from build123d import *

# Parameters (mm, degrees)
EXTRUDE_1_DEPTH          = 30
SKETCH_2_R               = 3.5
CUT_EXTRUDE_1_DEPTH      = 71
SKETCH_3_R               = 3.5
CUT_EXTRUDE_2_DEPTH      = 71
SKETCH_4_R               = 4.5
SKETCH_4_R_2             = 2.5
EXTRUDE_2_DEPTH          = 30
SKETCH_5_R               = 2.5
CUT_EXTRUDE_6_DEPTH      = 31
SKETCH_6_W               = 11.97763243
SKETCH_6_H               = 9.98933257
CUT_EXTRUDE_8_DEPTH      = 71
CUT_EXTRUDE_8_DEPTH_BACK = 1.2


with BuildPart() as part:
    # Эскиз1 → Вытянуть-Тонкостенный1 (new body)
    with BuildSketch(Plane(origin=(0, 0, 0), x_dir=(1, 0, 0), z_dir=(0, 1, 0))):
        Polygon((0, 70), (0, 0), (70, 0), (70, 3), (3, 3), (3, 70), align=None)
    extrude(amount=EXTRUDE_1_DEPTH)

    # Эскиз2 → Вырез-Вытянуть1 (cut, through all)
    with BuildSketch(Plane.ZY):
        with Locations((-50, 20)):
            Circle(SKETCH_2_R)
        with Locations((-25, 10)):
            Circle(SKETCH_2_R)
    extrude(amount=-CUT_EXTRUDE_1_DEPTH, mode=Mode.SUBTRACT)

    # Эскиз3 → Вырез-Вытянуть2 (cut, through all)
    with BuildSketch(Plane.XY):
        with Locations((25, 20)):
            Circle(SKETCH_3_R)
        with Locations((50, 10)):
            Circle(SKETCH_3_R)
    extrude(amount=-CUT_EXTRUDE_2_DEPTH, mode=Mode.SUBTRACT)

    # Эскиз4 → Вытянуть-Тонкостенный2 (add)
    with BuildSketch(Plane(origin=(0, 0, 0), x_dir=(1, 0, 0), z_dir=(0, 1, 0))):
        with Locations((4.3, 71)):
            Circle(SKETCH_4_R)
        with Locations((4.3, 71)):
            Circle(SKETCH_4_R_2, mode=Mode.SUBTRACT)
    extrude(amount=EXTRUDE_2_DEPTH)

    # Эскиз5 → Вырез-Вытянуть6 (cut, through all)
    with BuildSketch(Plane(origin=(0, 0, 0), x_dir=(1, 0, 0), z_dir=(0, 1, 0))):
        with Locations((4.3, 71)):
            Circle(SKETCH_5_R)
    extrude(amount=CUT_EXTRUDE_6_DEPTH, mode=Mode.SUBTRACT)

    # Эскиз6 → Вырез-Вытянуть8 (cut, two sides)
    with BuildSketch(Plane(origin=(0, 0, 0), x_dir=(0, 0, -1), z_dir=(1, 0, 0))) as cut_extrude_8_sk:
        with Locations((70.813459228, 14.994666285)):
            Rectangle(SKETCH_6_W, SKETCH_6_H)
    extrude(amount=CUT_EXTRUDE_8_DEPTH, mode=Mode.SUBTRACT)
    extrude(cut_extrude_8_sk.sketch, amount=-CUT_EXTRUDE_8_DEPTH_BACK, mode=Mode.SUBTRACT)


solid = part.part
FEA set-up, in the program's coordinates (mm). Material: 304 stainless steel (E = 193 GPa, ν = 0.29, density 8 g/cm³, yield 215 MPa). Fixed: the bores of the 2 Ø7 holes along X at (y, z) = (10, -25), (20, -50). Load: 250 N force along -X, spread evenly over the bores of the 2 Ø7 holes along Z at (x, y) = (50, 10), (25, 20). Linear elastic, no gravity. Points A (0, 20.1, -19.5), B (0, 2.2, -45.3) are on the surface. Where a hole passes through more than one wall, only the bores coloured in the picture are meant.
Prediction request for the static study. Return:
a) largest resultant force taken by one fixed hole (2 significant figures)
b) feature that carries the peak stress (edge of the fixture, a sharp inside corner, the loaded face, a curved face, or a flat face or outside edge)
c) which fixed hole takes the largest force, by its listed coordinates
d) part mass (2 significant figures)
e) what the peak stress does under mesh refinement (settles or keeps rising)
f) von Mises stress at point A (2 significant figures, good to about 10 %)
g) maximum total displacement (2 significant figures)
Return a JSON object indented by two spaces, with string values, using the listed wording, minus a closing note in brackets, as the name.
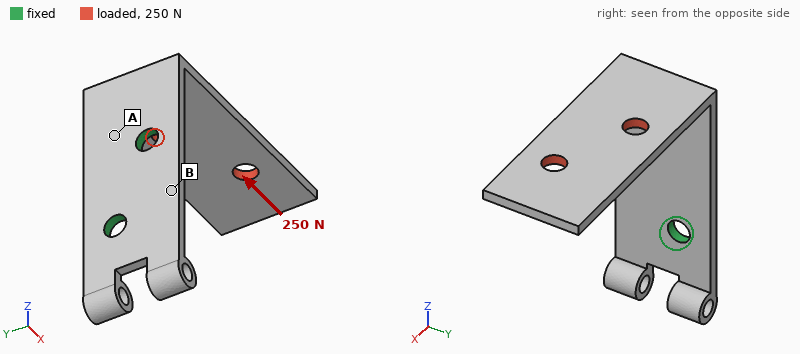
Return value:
{
  "largest resultant force taken by one fixed hole": "290 N",
  "feature that carries the peak stress": "edge of the fixture",
  "which fixed hole takes the largest force, by its listed coordinates": "(10, -25)",
  "part mass": "100 g",
  "what the peak stress does under mesh refinement": "keeps rising",
  "von Mises stress at point A": "74 MPa",
  "maximum total displacement": "0.34 mm"
}
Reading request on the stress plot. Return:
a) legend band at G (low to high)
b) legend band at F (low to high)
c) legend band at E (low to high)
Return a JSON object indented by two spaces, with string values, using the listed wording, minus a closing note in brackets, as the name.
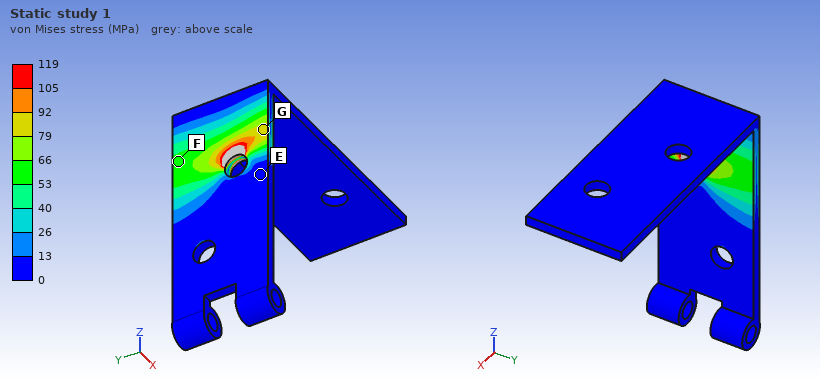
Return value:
{
  "legend band at G": "79 to 92 MPa",
  "legend band at F": "53 to 66 MPa",
  "legend band at E": "0 to 13 MPa"
}
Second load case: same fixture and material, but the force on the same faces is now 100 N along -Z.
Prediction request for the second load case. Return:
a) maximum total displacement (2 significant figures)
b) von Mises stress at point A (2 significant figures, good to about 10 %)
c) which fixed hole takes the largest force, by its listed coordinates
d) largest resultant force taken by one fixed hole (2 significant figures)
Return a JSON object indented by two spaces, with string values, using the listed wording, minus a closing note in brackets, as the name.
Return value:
{
  "maximum total displacement": "0.70 mm",
  "von Mises stress at point A": "62 MPa",
  "which fixed hole takes the largest force, by its listed coordinates": "(10, -25)",
  "largest resultant force taken by one fixed hole": "85 N"
}
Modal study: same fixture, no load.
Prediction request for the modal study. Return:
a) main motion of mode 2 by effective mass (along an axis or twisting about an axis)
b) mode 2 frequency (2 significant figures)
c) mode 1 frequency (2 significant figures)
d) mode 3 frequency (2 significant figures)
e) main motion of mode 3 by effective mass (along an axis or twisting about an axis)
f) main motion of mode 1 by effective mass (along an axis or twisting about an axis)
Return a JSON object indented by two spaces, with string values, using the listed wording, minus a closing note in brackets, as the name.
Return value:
{
  "main motion of mode 2 by effective mass": "along Y",
  "mode 2 frequency": "580 Hz",
  "mode 1 frequency": "340 Hz",
  "mode 3 frequency": "1600 Hz",
  "main motion of mode 3 by effective mass": "along X",
  "main motion of mode 1 by effective mass": "along Z"
}
